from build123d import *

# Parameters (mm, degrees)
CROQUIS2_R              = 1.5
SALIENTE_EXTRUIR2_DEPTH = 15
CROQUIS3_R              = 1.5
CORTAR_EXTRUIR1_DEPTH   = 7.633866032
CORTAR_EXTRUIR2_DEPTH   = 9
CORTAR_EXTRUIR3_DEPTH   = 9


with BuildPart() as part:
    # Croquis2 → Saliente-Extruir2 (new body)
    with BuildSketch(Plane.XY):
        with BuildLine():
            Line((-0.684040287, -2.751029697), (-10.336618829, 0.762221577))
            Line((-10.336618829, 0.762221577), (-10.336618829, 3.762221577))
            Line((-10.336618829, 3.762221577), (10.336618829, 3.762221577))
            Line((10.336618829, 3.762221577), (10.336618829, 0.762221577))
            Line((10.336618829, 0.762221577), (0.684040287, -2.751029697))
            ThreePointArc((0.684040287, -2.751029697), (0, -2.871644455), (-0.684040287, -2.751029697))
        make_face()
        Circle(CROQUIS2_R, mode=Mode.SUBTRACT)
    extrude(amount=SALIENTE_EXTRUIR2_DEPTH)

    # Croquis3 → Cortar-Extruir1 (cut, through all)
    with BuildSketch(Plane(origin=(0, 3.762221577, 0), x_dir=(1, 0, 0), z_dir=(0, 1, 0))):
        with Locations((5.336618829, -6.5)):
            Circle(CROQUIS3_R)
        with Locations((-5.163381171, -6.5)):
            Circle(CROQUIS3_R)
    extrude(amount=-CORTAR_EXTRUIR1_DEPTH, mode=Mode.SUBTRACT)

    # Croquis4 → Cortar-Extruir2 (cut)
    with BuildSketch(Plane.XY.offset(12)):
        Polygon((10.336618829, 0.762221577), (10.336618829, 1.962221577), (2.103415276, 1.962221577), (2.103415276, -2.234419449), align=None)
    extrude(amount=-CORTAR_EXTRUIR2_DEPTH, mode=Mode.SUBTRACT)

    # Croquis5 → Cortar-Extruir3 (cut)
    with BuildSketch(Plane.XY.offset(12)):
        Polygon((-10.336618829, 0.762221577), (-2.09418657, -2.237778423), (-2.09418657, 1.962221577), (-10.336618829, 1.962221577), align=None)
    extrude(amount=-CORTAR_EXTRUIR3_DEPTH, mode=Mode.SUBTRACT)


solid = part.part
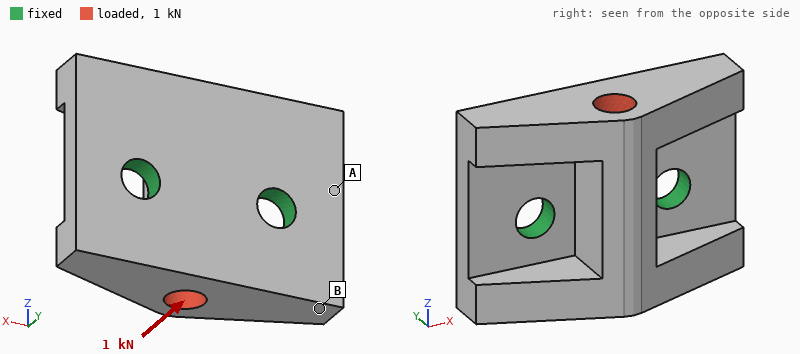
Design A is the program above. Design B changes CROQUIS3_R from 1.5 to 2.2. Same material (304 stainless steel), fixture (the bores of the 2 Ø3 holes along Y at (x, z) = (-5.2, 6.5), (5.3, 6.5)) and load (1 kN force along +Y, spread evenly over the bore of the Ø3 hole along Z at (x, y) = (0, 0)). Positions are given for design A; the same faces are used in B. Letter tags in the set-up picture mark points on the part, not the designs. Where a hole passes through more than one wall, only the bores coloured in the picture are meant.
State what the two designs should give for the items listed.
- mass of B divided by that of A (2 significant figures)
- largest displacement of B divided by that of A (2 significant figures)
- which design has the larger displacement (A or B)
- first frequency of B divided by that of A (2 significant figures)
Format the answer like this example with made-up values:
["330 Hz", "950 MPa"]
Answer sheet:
["0.97", "0.65", "A", "1.3"]
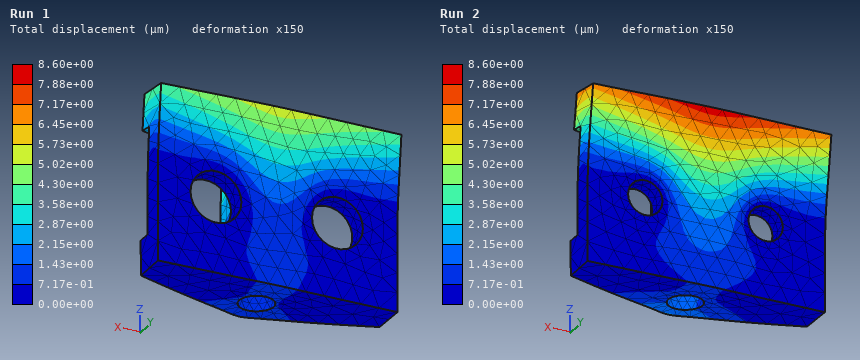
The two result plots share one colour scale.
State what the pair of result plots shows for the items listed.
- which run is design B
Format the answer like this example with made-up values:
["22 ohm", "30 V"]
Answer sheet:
["Run 1"]
